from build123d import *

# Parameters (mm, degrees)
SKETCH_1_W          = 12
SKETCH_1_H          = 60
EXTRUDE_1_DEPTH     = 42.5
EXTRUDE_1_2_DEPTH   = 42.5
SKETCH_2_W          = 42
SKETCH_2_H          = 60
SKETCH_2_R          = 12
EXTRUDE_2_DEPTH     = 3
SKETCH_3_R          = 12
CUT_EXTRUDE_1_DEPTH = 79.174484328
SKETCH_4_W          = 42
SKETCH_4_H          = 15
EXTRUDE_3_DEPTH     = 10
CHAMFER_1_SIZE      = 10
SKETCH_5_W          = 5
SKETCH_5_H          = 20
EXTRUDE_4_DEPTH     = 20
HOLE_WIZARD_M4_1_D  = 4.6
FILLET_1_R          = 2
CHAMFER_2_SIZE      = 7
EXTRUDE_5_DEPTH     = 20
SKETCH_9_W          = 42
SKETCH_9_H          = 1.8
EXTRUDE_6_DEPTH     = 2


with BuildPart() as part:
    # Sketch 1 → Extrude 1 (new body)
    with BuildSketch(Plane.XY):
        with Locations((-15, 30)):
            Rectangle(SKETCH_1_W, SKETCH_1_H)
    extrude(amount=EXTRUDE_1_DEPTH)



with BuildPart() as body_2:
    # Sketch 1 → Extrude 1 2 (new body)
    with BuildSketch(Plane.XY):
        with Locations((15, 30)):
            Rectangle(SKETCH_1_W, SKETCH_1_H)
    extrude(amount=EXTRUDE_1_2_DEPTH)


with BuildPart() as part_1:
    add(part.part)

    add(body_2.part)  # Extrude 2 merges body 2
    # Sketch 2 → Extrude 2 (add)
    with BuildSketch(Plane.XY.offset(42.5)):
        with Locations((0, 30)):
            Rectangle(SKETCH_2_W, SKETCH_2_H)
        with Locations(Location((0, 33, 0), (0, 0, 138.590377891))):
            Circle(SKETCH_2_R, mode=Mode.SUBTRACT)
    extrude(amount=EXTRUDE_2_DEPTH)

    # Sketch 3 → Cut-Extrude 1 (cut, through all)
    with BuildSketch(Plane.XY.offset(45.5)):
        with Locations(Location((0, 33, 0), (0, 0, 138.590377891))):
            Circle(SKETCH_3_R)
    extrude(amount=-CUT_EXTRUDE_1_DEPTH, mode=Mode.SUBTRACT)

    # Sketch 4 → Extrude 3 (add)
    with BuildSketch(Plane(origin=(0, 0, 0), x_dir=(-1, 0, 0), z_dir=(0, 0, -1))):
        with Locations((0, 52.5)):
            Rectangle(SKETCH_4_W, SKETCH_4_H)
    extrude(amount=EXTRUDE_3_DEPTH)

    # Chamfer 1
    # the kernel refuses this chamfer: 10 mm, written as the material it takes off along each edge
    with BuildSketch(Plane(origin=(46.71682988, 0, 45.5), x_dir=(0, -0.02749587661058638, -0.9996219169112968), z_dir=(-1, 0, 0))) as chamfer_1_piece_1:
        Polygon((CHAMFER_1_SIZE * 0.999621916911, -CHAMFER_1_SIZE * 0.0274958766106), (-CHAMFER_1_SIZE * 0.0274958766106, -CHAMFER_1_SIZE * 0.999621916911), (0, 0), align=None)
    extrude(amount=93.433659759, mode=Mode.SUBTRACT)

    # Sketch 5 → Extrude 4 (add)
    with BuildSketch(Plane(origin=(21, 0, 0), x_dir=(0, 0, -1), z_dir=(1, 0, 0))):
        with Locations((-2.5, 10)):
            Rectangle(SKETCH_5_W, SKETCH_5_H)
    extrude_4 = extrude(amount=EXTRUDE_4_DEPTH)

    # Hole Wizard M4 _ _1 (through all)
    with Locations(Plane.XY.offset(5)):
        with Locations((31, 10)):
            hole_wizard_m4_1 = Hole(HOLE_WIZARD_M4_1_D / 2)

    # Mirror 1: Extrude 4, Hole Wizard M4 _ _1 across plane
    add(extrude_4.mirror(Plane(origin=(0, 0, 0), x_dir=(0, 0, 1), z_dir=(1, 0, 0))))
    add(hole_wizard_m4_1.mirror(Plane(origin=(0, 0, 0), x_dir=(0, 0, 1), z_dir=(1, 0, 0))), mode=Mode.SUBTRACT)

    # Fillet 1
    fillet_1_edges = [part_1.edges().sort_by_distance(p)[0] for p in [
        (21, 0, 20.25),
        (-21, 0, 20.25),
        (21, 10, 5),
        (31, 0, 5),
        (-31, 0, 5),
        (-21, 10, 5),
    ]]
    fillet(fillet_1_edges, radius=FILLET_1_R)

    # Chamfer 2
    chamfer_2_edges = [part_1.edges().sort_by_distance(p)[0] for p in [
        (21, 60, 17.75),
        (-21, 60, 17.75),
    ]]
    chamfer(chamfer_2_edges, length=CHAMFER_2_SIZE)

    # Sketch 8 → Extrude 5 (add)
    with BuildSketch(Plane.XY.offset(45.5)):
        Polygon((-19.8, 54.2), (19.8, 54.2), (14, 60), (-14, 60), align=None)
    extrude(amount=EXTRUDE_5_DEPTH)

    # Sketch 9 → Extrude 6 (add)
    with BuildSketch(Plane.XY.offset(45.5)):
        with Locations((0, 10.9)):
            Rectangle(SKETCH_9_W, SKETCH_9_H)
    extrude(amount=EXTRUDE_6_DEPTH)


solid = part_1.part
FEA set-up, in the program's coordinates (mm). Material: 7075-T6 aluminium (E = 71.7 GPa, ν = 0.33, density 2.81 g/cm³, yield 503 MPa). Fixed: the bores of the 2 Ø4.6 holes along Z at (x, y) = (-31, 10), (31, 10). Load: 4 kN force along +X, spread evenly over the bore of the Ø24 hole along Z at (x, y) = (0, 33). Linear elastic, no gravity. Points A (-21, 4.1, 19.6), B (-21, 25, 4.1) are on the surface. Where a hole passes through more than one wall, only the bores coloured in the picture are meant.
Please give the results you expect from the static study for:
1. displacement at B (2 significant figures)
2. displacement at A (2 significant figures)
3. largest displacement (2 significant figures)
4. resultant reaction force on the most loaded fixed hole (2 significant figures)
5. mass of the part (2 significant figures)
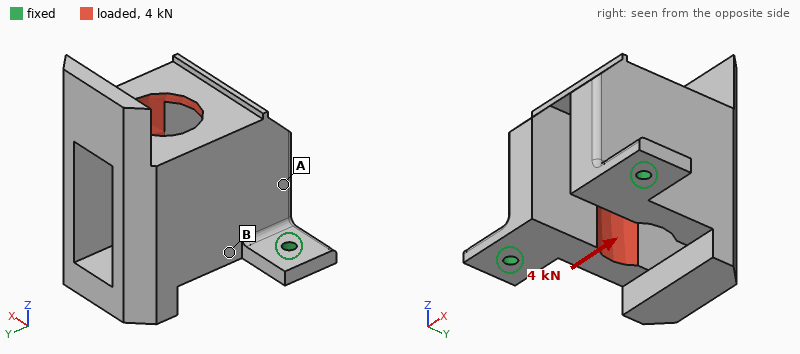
0.028 mm
0.050 mm
0.15 mm
2.9 kN
210 g
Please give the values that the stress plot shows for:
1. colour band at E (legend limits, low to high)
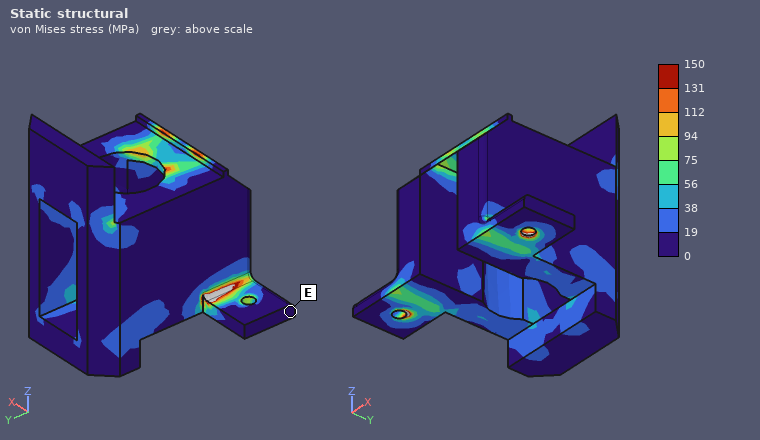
0 to 19 MPa
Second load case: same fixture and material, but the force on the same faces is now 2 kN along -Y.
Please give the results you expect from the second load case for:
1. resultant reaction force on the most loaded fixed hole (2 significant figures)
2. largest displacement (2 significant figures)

1.0 kN
0.77 mm
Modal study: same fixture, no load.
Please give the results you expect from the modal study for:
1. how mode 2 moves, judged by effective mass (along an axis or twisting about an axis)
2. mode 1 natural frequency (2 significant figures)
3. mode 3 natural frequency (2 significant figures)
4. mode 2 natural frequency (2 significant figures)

along X
620 Hz
3300 Hz
2300 Hz
